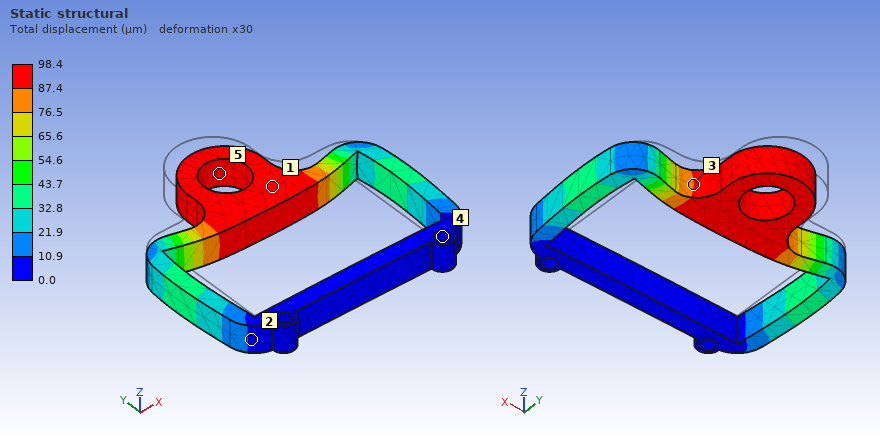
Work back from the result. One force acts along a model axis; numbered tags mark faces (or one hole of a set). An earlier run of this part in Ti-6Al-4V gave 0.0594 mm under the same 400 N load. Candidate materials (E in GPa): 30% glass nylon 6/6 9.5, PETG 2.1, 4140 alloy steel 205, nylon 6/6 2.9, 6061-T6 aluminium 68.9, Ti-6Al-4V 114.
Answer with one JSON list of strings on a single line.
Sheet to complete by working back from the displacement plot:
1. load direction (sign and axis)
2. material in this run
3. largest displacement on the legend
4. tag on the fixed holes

["-Y", "6061-T6 aluminium", "98.4 µm", "4"]
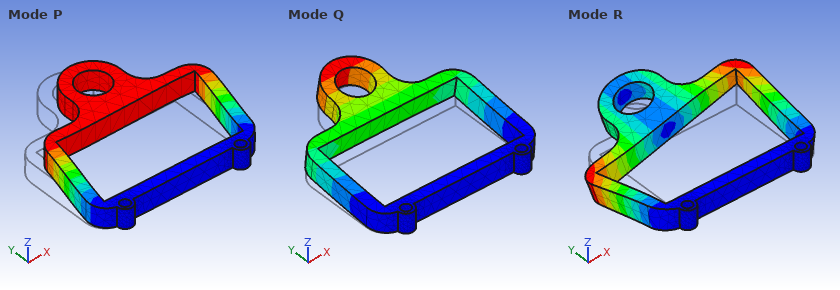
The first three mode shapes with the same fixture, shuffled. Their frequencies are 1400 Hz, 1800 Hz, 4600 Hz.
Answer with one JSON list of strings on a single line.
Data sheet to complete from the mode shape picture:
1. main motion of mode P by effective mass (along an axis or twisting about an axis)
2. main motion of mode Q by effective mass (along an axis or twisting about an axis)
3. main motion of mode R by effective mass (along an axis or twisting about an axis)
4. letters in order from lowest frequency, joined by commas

["along X", "along Z", "twisting about Y", "Q, P, R"]
